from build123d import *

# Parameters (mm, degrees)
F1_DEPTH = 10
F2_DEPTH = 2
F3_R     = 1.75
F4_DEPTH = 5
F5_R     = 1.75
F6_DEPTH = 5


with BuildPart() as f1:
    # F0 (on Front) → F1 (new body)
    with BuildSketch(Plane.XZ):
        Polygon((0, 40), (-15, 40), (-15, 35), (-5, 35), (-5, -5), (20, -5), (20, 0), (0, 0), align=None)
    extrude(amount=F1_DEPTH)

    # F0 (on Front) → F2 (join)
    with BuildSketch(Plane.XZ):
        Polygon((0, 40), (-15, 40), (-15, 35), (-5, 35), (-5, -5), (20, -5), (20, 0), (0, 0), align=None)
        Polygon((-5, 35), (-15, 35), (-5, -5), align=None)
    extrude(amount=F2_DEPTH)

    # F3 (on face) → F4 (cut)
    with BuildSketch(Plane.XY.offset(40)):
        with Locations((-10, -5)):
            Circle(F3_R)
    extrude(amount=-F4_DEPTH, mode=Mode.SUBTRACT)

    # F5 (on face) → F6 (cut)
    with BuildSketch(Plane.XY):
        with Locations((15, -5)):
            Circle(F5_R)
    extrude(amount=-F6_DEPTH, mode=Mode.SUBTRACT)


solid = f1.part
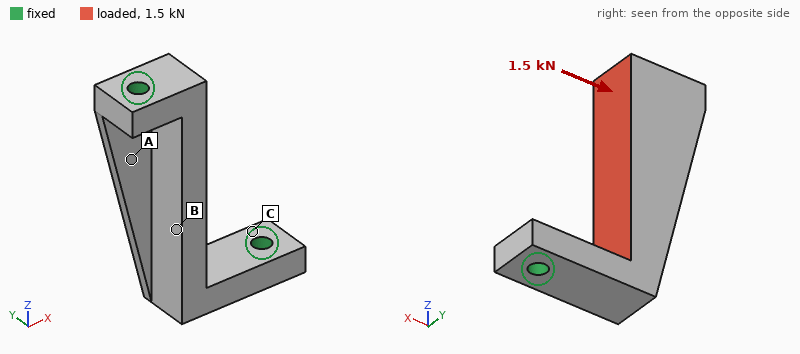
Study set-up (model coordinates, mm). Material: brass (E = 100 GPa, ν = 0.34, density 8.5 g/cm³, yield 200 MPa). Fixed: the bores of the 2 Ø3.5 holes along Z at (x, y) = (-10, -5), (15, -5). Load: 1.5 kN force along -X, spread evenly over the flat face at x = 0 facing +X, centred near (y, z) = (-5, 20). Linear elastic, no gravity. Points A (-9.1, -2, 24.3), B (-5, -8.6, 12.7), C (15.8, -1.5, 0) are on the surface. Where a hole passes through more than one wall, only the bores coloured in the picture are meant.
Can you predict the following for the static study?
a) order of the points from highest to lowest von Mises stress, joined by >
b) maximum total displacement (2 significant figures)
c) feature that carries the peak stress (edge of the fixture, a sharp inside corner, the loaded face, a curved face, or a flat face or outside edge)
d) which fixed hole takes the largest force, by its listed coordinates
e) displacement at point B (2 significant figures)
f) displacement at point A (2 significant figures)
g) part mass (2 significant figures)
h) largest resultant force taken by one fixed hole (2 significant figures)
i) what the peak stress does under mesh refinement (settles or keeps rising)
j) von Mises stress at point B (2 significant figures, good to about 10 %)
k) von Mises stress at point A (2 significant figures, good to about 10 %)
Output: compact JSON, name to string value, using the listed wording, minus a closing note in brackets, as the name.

{"order of the points from highest to lowest von Mises stress, joined by >": "B > A > C", "maximum total displacement": "35 µm", "feature that carries the peak stress": "edge of the fixture", "which fixed hole takes the largest force, by its listed coordinates": "(-10, -5)", "displacement at point B": "31 µm", "displacement at point A": "18 µm", "part mass": "34 g", "largest resultant force taken by one fixed hole": "880 N", "what the peak stress does under mesh refinement": "keeps rising", "von Mises stress at point B": "55 MPa", "von Mises stress at point A": "31 MPa"}
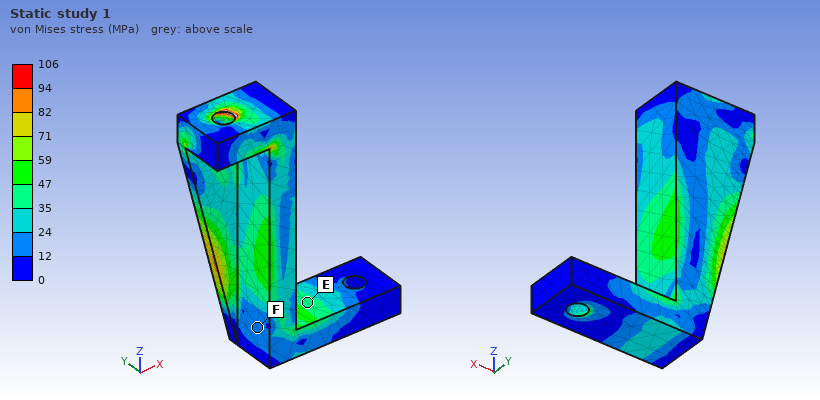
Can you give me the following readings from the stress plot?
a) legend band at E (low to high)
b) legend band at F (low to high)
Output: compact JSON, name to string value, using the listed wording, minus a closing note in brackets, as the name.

{"legend band at E": "35 to 47 MPa", "legend band at F": "12 to 24 MPa"}
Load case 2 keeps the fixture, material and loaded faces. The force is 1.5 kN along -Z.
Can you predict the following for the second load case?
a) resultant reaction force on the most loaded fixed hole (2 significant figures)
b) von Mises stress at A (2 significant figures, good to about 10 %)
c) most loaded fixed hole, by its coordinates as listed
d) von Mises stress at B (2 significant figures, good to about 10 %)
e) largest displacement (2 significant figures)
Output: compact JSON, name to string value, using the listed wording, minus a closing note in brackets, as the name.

{"resultant reaction force on the most loaded fixed hole": "1.4 kN", "von Mises stress at A": "34 MPa", "most loaded fixed hole, by its coordinates as listed": "(-10, -5)", "von Mises stress at B": "21 MPa", "largest displacement": "19 µm"}
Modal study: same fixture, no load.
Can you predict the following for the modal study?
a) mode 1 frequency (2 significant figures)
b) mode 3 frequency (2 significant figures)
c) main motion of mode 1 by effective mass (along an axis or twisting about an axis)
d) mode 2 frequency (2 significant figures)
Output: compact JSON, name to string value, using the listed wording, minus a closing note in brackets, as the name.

{"mode 1 frequency": "5900 Hz", "mode 3 frequency": "12 kHz", "main motion of mode 1 by effective mass": "along Y", "mode 2 frequency": "8300 Hz"}
